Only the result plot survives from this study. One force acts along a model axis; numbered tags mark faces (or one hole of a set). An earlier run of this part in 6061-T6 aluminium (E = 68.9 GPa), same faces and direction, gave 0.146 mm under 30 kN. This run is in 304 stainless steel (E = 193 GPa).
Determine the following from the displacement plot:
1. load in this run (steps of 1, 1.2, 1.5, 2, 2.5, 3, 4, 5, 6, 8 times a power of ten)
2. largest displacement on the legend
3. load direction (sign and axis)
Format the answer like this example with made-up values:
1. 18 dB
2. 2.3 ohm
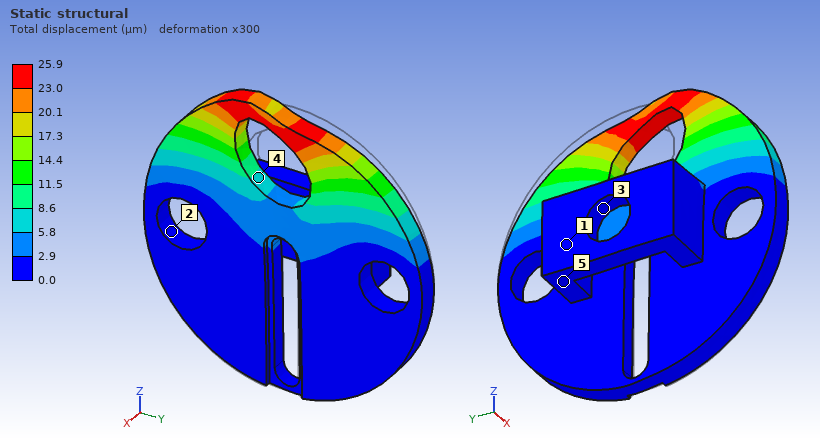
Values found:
1. 15 kN
2. 25.9 µm
3. -Y
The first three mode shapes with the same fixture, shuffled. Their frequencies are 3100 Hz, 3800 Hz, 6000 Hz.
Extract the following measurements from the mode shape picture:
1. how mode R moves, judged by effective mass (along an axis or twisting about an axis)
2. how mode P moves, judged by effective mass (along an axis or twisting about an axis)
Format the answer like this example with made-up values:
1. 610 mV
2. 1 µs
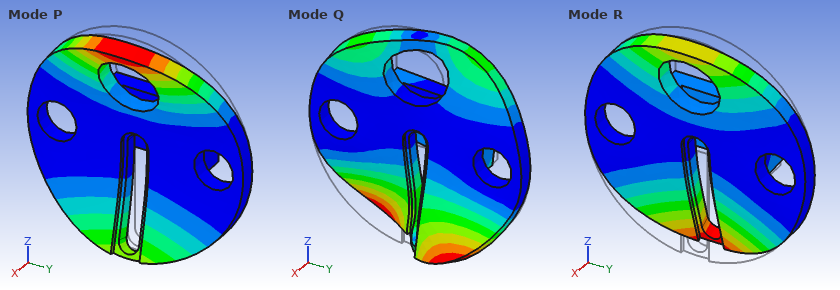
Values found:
1. twisting about Y
2. along X
